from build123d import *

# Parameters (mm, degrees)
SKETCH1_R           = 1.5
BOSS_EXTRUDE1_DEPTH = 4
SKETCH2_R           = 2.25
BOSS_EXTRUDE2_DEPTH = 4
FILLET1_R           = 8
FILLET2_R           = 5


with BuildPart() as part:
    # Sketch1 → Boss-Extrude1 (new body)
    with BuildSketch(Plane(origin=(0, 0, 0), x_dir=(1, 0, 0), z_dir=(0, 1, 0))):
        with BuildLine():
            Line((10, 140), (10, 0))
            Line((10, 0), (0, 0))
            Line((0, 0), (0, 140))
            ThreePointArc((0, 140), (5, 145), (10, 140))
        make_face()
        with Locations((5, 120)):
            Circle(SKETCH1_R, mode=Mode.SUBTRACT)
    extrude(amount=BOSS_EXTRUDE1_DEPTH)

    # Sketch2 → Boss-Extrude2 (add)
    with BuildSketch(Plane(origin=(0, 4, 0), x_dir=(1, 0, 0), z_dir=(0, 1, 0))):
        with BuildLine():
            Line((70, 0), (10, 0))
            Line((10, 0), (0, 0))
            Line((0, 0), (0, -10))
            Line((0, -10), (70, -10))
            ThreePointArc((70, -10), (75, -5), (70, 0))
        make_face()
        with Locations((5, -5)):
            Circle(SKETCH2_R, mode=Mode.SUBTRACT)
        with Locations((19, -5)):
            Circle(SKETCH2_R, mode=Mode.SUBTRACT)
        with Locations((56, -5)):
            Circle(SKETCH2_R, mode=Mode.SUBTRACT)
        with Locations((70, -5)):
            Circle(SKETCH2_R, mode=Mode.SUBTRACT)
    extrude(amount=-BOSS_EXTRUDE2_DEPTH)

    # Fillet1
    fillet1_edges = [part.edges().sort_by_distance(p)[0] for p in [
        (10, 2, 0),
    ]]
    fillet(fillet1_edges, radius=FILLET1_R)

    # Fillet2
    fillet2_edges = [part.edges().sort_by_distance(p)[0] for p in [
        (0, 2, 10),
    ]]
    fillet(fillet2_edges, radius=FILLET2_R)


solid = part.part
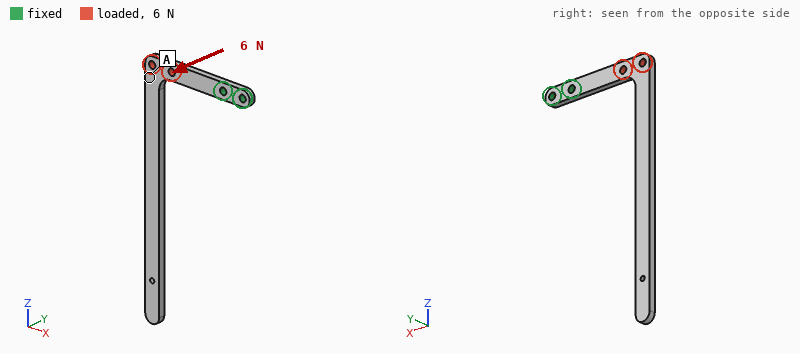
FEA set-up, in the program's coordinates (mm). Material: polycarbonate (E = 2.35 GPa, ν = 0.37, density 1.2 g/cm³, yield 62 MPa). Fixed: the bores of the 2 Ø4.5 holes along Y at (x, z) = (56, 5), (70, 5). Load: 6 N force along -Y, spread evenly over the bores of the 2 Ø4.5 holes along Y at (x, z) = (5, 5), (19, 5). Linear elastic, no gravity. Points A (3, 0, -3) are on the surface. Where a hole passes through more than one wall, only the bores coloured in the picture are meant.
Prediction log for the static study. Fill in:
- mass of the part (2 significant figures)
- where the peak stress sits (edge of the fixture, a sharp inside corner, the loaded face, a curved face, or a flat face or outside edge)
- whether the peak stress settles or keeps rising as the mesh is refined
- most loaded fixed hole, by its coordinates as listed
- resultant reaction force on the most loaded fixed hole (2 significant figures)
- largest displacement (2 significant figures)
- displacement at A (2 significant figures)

10 g
edge of the fixture
keeps rising
(56, 5)
6.7 N
1.8 mm
1.7 mm
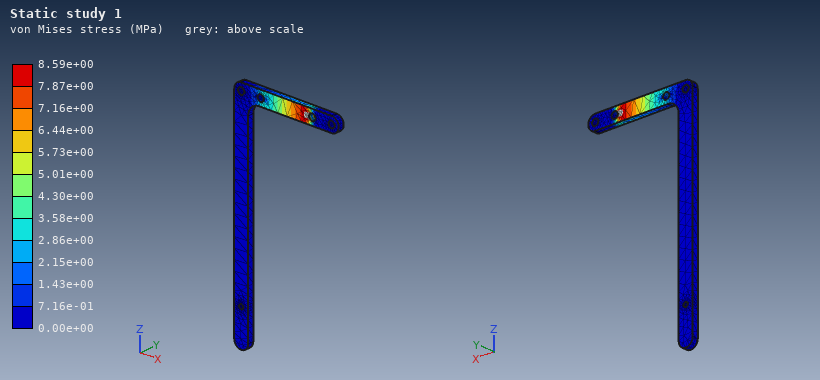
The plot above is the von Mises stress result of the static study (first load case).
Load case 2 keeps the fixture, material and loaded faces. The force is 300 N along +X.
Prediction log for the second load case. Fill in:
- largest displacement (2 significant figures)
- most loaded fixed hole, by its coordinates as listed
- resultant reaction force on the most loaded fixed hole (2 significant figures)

0.16 mm
(56, 5)
290 N
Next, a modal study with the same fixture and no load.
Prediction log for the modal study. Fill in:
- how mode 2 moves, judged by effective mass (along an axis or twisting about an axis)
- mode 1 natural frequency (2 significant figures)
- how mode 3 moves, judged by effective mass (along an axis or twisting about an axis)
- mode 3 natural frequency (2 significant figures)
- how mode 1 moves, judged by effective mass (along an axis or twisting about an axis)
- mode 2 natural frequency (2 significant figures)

along X
27 Hz
along Y
140 Hz
along Y
67 Hz
